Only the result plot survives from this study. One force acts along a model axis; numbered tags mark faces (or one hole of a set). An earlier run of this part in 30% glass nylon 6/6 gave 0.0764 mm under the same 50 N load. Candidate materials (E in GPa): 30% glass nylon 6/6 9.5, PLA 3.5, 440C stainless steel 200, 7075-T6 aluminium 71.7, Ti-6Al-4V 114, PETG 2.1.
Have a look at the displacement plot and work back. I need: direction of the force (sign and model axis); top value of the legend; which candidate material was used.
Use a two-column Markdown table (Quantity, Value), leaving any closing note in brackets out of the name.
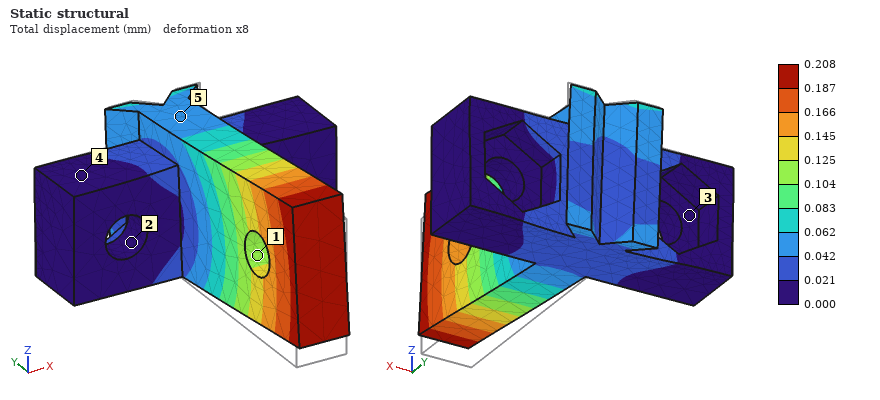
| Quantity | Value |
|---|---|
| direction of the force | +Z |
| top value of the legend | 0.208 mm |
| which candidate material was used | PLA |
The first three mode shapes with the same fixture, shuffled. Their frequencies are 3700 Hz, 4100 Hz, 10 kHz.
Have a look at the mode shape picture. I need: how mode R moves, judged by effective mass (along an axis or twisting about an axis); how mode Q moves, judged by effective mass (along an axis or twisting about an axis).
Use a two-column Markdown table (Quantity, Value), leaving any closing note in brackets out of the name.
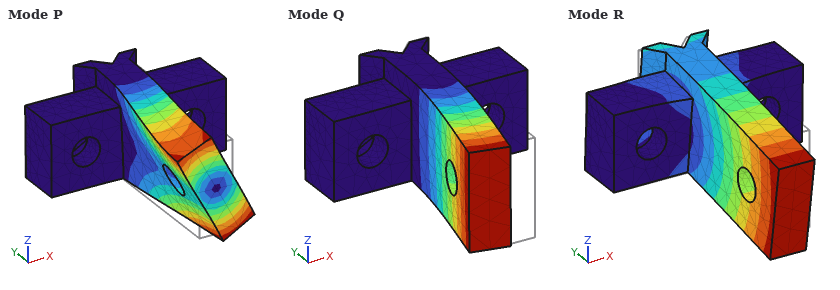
| Quantity | Value |
|---|---|
| how mode R moves, judged by effective mass | along Z |
| how mode Q moves, judged by effective mass | along X |
